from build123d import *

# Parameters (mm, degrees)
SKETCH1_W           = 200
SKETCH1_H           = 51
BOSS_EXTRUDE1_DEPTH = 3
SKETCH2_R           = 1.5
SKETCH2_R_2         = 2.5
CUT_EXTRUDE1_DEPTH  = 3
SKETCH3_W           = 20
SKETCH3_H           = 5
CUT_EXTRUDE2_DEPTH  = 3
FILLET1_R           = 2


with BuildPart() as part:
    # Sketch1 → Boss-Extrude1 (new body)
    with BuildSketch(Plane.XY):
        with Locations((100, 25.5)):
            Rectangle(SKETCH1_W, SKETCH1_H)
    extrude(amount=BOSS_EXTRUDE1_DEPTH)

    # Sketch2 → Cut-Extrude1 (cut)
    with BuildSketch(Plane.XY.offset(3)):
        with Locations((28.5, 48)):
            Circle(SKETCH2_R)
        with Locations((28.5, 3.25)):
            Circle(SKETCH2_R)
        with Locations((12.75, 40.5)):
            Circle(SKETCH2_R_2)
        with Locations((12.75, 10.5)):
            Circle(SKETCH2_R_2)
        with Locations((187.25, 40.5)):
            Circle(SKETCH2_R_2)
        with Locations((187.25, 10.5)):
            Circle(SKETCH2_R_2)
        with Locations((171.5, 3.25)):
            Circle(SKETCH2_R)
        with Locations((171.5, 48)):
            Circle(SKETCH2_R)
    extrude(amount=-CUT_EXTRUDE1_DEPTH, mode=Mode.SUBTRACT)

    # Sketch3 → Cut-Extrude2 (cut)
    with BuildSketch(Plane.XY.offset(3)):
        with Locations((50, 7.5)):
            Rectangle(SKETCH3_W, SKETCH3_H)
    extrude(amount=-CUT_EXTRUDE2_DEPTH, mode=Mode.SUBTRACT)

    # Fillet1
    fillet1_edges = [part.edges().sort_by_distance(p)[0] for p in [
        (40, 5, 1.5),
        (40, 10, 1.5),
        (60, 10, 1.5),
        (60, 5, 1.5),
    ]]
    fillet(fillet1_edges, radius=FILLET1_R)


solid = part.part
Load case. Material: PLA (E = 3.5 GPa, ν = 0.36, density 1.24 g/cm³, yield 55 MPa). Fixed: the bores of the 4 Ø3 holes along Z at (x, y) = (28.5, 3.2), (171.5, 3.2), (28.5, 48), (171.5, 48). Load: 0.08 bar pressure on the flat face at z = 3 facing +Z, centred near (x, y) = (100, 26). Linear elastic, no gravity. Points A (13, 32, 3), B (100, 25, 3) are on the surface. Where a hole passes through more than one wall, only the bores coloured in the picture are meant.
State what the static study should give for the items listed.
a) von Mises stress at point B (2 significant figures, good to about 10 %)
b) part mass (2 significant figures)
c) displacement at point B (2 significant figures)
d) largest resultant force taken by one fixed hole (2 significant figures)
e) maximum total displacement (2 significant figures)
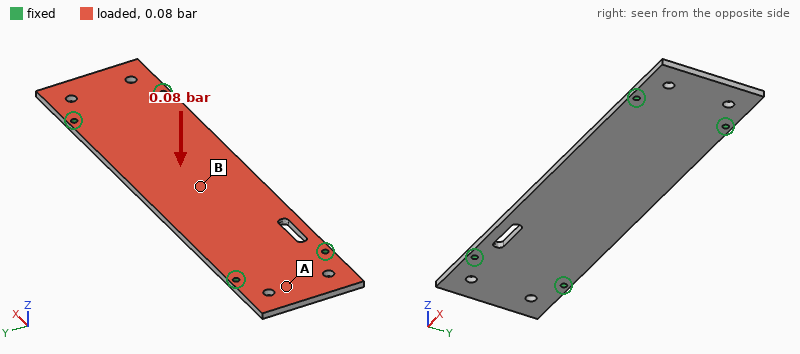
4.6 MPa
37 g
1.3 mm
20 N
1.3 mm
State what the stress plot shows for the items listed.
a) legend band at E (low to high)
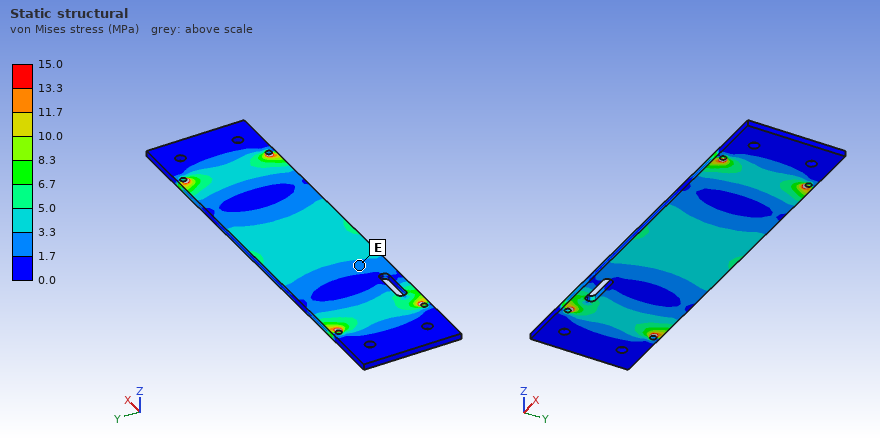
1.7 to 3.3 MPa
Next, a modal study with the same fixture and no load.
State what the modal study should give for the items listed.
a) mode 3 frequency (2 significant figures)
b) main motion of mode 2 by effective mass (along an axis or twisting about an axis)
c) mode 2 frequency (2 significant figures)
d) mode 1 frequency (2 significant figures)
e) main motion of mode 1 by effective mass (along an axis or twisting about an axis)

620 Hz
twisting about X
510 Hz
230 Hz
along Z
